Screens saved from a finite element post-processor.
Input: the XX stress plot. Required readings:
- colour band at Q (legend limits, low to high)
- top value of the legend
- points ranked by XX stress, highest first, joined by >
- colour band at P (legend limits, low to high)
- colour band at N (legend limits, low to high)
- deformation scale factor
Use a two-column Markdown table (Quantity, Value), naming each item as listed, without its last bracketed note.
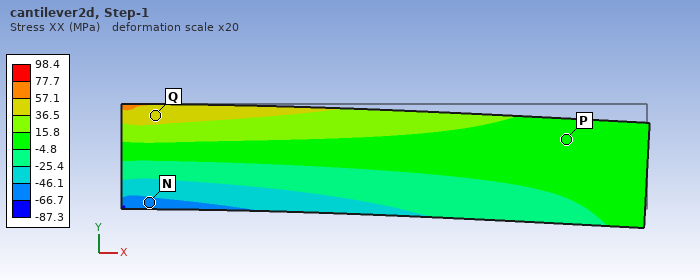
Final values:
| Quantity | Value |
|---|---|
| colour band at Q | 36.5 to 57.1 MPa |
| top value of the legend | 98.4 MPa |
| points ranked by XX stress, highest first, joined by > | Q > P > N |
| colour band at P | -4.8 to 15.8 MPa |
| colour band at N | -66.7 to -46.1 MPa |
| deformation scale factor | 20 |
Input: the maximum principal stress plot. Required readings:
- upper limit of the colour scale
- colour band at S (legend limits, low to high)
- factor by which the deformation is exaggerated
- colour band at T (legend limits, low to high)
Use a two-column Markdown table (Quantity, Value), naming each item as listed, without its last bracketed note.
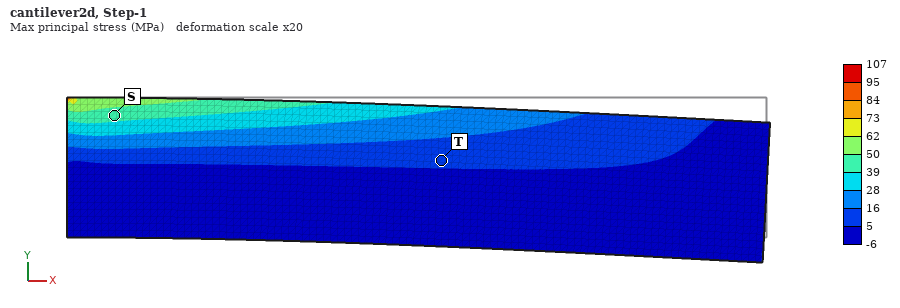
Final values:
| Quantity | Value |
|---|---|
| upper limit of the colour scale | 107 MPa |
| colour band at S | 39 to 50 MPa |
| factor by which the deformation is exaggerated | 20 |
| colour band at T | 5 to 16 MPa |
